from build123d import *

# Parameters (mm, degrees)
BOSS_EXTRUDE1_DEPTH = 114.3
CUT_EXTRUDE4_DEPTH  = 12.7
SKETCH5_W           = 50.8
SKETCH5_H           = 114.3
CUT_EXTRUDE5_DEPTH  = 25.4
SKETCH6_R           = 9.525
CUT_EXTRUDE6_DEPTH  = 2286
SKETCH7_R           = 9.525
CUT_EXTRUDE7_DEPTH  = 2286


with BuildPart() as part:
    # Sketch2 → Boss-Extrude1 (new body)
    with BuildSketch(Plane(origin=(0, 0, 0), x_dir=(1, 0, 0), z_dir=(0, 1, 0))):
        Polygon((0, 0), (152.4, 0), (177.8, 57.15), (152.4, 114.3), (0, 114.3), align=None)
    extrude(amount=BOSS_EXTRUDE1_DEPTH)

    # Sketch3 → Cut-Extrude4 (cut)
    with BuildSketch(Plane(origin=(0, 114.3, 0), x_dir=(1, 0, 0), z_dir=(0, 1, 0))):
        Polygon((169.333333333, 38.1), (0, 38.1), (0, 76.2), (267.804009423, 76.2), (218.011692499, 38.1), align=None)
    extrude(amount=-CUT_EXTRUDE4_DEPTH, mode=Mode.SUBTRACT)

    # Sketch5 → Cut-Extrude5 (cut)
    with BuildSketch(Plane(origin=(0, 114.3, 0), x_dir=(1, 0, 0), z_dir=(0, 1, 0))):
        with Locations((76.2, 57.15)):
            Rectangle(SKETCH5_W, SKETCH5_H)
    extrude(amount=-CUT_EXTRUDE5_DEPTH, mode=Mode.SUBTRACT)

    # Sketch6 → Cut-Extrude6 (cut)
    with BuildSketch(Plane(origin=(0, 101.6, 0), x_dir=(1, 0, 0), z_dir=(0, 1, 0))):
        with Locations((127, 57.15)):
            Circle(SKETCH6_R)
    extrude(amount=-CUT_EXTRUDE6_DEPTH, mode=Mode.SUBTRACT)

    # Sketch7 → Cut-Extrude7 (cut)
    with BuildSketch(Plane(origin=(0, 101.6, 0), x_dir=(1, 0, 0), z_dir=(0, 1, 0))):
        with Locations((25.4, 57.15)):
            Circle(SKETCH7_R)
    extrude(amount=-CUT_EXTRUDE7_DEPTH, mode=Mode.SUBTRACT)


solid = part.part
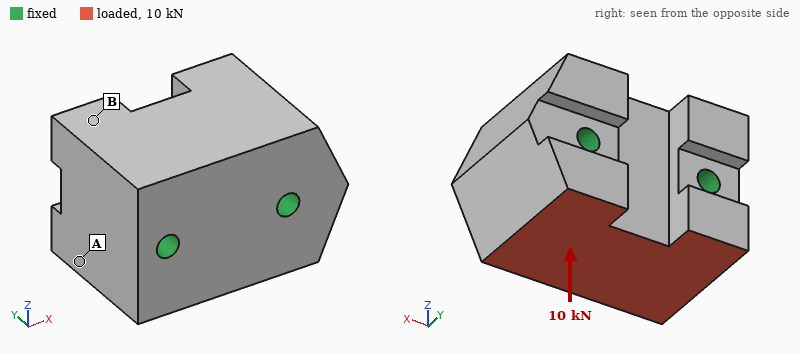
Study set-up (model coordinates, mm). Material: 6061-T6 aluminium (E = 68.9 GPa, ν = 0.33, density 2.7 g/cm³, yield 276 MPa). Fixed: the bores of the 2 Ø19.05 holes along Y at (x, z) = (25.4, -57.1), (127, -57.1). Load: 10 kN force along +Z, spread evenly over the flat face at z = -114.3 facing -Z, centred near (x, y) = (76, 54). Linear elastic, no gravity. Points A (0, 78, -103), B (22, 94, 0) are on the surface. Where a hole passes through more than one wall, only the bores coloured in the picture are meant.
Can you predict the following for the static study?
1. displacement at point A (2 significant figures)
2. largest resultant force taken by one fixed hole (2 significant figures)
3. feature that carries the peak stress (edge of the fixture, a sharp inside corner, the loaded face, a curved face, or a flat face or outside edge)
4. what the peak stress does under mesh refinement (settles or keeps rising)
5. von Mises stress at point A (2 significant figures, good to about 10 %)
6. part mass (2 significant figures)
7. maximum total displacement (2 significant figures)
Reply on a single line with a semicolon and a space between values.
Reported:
0.54 µm; 5.1 kN; edge of the fixture; keeps rising; 0.70 MPa; 5.1 kg; 1.0 µm
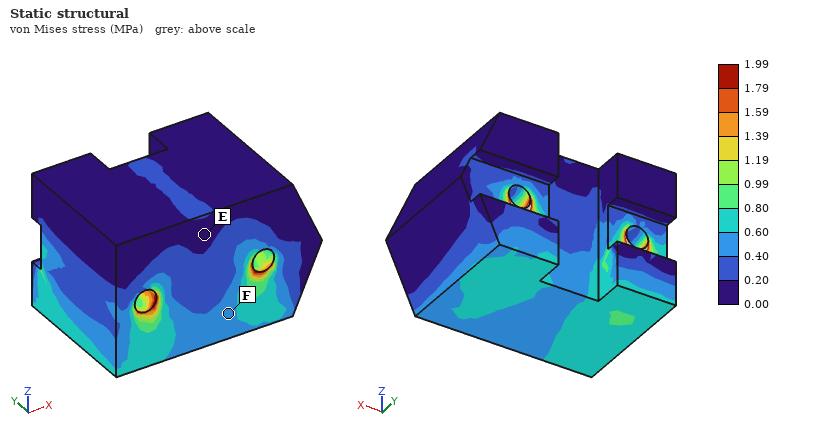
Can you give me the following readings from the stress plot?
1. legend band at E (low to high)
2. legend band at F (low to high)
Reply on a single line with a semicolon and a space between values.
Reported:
0.00 to 0.20 MPa; 0.40 to 0.60 MPa
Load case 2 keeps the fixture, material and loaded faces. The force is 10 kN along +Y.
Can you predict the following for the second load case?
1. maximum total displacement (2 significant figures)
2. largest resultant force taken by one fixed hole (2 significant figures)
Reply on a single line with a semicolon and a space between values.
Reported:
4.0 µm; 5.0 kN
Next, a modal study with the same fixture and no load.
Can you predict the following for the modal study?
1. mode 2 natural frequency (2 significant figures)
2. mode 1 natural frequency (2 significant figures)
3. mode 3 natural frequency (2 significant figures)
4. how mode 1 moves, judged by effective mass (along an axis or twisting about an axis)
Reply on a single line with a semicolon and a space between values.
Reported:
9300 Hz; 9000 Hz; 9700 Hz; twisting about X
